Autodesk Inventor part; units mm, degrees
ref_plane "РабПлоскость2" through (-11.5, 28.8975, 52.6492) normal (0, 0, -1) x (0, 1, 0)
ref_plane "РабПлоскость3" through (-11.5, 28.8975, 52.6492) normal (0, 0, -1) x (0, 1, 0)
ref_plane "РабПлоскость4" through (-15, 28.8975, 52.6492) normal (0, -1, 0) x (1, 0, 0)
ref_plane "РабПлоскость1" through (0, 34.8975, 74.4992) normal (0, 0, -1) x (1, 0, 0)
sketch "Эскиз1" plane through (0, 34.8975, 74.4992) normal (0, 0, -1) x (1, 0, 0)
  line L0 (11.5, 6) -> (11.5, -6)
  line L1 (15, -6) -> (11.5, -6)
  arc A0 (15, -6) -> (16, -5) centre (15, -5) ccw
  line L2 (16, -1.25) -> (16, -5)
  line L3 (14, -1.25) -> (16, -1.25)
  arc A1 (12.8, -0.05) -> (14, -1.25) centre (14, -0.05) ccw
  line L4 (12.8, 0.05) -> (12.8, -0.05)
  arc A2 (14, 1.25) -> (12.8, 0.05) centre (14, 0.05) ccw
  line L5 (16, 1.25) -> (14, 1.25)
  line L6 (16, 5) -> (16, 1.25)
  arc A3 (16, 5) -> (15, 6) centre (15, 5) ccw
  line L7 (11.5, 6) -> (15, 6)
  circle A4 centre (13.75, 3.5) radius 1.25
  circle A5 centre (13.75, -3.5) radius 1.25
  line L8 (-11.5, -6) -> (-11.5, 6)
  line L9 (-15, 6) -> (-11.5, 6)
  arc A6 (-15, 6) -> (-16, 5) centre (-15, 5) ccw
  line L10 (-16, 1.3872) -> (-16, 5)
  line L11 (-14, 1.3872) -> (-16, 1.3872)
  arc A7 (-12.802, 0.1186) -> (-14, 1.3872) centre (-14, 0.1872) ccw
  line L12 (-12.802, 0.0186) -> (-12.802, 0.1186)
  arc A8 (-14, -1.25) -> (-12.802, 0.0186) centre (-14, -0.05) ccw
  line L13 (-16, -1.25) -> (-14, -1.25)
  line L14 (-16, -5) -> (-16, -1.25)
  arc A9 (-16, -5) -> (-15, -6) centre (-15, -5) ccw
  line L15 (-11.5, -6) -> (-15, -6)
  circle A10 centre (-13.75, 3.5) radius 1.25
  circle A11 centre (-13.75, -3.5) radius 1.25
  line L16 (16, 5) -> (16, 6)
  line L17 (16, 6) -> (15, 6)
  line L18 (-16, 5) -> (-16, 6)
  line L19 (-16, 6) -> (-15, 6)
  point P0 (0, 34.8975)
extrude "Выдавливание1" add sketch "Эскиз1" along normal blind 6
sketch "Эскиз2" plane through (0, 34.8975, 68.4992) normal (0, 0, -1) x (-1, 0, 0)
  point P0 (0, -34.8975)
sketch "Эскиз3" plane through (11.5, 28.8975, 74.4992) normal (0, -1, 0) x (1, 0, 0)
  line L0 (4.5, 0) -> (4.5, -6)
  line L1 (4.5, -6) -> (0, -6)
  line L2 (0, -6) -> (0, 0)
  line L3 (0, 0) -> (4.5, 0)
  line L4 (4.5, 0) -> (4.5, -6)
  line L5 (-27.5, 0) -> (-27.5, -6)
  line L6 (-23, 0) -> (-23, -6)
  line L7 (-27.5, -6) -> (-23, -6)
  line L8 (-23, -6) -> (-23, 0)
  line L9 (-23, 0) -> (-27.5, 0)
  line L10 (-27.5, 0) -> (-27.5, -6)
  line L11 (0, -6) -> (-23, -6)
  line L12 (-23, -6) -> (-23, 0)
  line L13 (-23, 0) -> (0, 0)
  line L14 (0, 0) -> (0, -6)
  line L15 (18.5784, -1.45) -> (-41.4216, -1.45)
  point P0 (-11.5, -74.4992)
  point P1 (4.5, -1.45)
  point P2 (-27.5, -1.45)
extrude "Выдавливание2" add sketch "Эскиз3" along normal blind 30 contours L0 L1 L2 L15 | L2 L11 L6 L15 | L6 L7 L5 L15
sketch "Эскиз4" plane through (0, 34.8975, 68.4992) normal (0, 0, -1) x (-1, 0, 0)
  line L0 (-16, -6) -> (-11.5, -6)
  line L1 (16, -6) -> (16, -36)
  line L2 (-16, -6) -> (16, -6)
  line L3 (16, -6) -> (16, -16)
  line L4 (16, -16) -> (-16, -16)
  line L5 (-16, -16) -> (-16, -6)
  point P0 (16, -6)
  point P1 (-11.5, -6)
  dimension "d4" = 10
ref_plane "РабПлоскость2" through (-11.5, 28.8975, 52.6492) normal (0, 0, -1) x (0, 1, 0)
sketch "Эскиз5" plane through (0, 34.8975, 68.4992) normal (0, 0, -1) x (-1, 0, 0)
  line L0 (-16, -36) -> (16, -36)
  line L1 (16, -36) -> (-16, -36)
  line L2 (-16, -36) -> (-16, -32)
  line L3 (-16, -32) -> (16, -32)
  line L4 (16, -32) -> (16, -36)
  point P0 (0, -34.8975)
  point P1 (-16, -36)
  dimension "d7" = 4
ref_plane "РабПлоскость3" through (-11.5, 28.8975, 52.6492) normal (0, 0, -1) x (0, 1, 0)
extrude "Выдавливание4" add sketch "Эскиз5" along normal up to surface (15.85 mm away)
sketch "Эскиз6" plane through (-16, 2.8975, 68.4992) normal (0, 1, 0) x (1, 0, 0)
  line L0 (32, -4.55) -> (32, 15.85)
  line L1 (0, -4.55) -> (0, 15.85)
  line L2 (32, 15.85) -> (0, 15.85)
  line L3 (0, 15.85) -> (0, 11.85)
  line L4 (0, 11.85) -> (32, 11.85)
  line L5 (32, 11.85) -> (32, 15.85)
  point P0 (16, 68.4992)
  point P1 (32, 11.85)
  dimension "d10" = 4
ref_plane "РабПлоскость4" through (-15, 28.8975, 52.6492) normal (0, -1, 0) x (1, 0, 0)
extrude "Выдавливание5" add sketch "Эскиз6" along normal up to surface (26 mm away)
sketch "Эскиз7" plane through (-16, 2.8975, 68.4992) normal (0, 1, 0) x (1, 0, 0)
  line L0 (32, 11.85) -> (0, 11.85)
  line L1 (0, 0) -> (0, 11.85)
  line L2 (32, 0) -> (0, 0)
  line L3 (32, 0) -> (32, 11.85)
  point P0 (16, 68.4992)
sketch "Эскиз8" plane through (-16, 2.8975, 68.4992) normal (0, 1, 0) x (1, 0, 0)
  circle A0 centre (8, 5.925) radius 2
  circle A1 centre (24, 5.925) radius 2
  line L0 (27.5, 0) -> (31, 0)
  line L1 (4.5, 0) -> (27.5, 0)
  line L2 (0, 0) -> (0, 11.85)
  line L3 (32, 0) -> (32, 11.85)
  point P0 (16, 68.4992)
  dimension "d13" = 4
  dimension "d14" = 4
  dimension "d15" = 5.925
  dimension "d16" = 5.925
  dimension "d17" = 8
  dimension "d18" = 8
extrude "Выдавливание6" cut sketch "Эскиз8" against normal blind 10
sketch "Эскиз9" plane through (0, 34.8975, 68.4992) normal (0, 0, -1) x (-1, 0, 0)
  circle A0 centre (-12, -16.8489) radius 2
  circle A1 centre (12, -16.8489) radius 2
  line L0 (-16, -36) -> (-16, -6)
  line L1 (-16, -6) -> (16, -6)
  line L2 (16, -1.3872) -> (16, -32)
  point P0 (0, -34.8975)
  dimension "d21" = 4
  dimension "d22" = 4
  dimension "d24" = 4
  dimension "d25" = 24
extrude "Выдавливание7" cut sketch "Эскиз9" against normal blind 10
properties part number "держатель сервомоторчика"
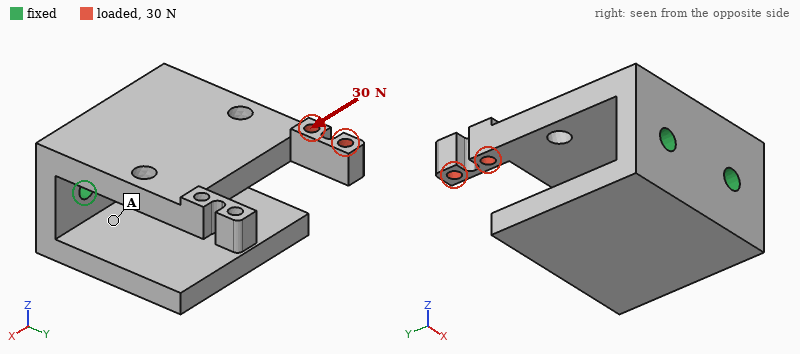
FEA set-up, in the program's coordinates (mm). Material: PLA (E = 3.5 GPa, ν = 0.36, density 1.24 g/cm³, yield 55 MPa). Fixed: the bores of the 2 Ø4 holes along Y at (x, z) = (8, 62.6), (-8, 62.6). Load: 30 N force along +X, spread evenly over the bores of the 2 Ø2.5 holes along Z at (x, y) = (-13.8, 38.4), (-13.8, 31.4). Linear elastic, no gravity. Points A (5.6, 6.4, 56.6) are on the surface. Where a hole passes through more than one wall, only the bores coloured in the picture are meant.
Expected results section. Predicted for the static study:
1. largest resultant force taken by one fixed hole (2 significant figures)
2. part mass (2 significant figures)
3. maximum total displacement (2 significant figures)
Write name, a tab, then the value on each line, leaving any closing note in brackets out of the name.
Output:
largest resultant force taken by one fixed hole	55 N
part mass	12 g
maximum total displacement	0.53 mm
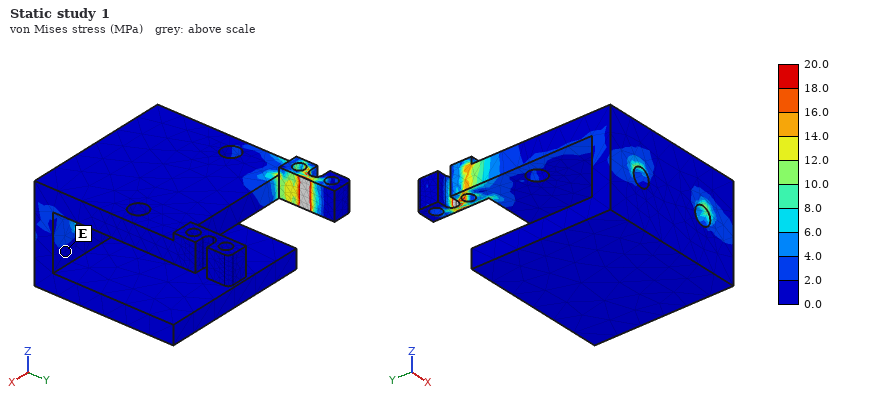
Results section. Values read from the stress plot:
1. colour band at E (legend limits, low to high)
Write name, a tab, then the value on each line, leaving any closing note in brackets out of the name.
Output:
colour band at E	0.0 to 2.0 MPa
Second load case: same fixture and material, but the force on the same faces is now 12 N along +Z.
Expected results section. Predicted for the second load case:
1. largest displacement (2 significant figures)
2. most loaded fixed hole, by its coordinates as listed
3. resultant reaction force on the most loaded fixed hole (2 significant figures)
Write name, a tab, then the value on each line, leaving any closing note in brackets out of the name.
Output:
largest displacement	0.58 mm
most loaded fixed hole, by its coordinates as listed	(-8, 62.6)
resultant reaction force on the most loaded fixed hole	15 N
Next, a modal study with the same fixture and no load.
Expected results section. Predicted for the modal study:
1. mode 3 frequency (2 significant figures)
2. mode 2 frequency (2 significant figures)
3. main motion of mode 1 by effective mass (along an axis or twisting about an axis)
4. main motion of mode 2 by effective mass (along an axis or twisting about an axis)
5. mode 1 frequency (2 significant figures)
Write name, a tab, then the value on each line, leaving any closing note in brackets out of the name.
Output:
mode 3 frequency	1800 Hz
mode 2 frequency	1000 Hz
main motion of mode 1 by effective mass	along Z
main motion of mode 2 by effective mass	along Z
mode 1 frequency	820 Hz
